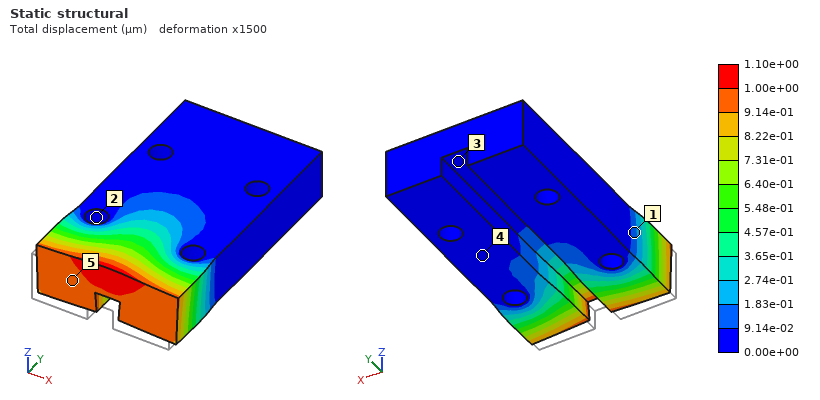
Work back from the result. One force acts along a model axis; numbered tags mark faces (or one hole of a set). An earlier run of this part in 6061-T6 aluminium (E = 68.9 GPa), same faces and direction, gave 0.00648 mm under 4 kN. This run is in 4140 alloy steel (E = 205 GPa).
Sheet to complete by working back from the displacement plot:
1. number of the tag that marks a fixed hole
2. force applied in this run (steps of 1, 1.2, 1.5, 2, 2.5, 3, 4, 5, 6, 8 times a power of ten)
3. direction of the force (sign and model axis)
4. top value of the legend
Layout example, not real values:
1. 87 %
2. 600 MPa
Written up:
1. 2
2. 2 kN
3. +Y
4. 1.10e+00 µm
